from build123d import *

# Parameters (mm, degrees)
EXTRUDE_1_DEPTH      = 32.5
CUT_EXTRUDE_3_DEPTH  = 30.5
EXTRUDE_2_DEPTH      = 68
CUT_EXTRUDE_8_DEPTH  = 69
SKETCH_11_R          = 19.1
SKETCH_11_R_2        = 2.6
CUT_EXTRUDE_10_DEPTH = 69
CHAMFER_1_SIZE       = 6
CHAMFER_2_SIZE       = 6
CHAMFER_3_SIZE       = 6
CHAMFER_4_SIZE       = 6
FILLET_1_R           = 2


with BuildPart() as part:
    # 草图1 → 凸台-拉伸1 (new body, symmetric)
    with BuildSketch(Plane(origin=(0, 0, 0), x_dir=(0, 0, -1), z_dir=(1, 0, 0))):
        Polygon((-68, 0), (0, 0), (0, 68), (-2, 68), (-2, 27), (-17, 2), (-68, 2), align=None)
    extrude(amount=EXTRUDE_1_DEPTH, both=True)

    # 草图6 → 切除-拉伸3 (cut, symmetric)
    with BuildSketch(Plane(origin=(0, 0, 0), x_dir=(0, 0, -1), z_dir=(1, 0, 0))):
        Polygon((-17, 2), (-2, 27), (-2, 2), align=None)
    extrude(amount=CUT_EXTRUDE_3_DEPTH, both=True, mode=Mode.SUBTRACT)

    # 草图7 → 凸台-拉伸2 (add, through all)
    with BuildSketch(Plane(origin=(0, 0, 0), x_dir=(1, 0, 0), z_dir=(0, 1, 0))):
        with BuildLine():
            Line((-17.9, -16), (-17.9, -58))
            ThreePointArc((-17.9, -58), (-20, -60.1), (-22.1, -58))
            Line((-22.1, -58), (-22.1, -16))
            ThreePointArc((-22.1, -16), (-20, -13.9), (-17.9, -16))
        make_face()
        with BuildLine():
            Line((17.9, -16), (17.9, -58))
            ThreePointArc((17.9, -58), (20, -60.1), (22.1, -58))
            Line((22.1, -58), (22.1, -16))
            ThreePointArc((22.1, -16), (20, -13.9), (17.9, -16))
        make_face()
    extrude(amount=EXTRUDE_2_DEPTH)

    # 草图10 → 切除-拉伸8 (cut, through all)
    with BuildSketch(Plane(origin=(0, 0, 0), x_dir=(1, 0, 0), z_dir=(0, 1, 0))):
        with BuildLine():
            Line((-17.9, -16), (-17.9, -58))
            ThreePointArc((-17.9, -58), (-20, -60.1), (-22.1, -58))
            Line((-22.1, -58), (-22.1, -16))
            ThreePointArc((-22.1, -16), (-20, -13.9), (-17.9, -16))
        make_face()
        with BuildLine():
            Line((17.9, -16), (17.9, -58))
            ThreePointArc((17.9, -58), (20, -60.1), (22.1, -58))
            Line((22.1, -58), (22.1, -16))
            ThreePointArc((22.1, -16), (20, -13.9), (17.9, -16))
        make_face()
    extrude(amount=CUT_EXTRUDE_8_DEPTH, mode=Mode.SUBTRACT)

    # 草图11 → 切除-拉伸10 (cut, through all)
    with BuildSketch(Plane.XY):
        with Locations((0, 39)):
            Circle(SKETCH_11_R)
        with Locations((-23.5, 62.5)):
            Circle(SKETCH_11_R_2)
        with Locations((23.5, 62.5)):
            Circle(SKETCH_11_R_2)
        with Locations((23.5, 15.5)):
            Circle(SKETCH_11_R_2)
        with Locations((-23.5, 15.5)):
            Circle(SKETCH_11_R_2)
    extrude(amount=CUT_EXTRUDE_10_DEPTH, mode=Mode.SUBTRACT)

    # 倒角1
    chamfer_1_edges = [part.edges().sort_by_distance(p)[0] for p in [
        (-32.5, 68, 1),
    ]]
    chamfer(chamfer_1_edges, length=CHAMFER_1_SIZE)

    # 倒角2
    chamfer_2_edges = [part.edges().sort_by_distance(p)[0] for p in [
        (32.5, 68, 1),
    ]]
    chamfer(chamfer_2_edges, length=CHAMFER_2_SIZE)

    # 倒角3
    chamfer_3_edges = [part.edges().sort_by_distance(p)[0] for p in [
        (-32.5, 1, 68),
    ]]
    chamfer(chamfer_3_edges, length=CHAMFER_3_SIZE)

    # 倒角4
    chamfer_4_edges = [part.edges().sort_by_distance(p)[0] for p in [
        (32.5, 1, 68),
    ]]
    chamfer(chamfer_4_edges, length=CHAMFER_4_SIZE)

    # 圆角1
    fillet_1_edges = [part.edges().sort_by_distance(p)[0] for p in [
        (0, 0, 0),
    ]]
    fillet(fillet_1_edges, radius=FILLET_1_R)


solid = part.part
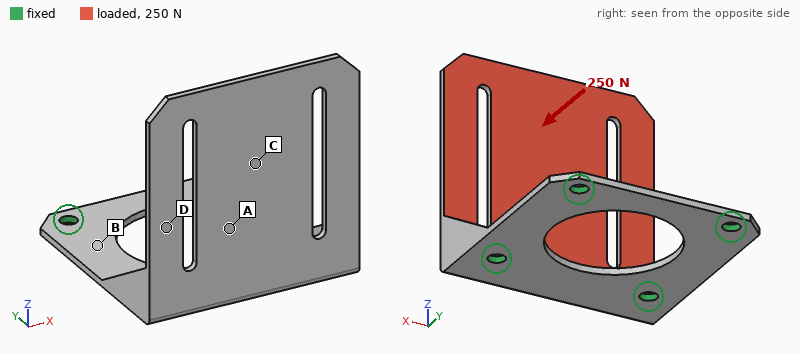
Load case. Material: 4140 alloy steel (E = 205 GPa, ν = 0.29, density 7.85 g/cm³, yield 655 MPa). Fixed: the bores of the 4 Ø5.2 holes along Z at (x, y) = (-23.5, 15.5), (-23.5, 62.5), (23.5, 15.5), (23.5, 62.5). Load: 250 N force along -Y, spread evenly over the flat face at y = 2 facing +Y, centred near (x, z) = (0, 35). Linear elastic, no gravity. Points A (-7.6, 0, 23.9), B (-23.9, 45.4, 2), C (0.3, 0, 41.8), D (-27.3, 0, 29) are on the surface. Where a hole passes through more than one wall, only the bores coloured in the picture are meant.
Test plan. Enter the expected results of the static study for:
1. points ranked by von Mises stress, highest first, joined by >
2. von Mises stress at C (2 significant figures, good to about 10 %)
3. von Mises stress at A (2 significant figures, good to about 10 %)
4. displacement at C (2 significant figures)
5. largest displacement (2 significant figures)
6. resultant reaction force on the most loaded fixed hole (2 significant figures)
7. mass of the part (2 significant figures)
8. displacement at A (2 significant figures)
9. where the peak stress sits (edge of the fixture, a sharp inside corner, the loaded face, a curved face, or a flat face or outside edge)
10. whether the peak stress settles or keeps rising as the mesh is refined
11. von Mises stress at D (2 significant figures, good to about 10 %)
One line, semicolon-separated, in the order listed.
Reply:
D > A > C > B; 36 MPa; 72 MPa; 0.54 mm; 1.1 mm; 150 N; 120 g; 0.24 mm; a sharp inside corner; keeps rising; 120 MPa
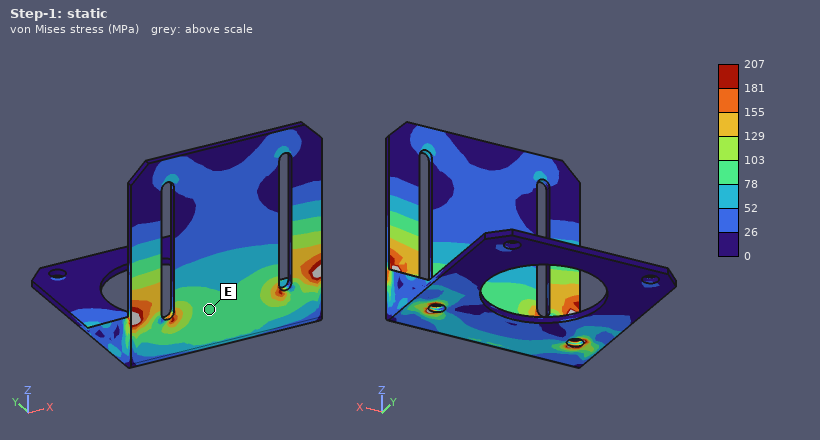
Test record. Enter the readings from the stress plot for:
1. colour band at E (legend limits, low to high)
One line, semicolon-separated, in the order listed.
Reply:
78 to 103 MPa
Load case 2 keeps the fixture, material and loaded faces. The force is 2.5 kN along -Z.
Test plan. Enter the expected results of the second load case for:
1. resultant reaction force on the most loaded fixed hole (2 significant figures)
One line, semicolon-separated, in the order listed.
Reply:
1.3 kN
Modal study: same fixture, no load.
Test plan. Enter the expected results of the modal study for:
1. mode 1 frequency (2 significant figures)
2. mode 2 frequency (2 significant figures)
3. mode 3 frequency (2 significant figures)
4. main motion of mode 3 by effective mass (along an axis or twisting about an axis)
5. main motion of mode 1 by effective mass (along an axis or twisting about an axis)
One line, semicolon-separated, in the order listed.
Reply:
390 Hz; 1000 Hz; 1700 Hz; along X; along Y
